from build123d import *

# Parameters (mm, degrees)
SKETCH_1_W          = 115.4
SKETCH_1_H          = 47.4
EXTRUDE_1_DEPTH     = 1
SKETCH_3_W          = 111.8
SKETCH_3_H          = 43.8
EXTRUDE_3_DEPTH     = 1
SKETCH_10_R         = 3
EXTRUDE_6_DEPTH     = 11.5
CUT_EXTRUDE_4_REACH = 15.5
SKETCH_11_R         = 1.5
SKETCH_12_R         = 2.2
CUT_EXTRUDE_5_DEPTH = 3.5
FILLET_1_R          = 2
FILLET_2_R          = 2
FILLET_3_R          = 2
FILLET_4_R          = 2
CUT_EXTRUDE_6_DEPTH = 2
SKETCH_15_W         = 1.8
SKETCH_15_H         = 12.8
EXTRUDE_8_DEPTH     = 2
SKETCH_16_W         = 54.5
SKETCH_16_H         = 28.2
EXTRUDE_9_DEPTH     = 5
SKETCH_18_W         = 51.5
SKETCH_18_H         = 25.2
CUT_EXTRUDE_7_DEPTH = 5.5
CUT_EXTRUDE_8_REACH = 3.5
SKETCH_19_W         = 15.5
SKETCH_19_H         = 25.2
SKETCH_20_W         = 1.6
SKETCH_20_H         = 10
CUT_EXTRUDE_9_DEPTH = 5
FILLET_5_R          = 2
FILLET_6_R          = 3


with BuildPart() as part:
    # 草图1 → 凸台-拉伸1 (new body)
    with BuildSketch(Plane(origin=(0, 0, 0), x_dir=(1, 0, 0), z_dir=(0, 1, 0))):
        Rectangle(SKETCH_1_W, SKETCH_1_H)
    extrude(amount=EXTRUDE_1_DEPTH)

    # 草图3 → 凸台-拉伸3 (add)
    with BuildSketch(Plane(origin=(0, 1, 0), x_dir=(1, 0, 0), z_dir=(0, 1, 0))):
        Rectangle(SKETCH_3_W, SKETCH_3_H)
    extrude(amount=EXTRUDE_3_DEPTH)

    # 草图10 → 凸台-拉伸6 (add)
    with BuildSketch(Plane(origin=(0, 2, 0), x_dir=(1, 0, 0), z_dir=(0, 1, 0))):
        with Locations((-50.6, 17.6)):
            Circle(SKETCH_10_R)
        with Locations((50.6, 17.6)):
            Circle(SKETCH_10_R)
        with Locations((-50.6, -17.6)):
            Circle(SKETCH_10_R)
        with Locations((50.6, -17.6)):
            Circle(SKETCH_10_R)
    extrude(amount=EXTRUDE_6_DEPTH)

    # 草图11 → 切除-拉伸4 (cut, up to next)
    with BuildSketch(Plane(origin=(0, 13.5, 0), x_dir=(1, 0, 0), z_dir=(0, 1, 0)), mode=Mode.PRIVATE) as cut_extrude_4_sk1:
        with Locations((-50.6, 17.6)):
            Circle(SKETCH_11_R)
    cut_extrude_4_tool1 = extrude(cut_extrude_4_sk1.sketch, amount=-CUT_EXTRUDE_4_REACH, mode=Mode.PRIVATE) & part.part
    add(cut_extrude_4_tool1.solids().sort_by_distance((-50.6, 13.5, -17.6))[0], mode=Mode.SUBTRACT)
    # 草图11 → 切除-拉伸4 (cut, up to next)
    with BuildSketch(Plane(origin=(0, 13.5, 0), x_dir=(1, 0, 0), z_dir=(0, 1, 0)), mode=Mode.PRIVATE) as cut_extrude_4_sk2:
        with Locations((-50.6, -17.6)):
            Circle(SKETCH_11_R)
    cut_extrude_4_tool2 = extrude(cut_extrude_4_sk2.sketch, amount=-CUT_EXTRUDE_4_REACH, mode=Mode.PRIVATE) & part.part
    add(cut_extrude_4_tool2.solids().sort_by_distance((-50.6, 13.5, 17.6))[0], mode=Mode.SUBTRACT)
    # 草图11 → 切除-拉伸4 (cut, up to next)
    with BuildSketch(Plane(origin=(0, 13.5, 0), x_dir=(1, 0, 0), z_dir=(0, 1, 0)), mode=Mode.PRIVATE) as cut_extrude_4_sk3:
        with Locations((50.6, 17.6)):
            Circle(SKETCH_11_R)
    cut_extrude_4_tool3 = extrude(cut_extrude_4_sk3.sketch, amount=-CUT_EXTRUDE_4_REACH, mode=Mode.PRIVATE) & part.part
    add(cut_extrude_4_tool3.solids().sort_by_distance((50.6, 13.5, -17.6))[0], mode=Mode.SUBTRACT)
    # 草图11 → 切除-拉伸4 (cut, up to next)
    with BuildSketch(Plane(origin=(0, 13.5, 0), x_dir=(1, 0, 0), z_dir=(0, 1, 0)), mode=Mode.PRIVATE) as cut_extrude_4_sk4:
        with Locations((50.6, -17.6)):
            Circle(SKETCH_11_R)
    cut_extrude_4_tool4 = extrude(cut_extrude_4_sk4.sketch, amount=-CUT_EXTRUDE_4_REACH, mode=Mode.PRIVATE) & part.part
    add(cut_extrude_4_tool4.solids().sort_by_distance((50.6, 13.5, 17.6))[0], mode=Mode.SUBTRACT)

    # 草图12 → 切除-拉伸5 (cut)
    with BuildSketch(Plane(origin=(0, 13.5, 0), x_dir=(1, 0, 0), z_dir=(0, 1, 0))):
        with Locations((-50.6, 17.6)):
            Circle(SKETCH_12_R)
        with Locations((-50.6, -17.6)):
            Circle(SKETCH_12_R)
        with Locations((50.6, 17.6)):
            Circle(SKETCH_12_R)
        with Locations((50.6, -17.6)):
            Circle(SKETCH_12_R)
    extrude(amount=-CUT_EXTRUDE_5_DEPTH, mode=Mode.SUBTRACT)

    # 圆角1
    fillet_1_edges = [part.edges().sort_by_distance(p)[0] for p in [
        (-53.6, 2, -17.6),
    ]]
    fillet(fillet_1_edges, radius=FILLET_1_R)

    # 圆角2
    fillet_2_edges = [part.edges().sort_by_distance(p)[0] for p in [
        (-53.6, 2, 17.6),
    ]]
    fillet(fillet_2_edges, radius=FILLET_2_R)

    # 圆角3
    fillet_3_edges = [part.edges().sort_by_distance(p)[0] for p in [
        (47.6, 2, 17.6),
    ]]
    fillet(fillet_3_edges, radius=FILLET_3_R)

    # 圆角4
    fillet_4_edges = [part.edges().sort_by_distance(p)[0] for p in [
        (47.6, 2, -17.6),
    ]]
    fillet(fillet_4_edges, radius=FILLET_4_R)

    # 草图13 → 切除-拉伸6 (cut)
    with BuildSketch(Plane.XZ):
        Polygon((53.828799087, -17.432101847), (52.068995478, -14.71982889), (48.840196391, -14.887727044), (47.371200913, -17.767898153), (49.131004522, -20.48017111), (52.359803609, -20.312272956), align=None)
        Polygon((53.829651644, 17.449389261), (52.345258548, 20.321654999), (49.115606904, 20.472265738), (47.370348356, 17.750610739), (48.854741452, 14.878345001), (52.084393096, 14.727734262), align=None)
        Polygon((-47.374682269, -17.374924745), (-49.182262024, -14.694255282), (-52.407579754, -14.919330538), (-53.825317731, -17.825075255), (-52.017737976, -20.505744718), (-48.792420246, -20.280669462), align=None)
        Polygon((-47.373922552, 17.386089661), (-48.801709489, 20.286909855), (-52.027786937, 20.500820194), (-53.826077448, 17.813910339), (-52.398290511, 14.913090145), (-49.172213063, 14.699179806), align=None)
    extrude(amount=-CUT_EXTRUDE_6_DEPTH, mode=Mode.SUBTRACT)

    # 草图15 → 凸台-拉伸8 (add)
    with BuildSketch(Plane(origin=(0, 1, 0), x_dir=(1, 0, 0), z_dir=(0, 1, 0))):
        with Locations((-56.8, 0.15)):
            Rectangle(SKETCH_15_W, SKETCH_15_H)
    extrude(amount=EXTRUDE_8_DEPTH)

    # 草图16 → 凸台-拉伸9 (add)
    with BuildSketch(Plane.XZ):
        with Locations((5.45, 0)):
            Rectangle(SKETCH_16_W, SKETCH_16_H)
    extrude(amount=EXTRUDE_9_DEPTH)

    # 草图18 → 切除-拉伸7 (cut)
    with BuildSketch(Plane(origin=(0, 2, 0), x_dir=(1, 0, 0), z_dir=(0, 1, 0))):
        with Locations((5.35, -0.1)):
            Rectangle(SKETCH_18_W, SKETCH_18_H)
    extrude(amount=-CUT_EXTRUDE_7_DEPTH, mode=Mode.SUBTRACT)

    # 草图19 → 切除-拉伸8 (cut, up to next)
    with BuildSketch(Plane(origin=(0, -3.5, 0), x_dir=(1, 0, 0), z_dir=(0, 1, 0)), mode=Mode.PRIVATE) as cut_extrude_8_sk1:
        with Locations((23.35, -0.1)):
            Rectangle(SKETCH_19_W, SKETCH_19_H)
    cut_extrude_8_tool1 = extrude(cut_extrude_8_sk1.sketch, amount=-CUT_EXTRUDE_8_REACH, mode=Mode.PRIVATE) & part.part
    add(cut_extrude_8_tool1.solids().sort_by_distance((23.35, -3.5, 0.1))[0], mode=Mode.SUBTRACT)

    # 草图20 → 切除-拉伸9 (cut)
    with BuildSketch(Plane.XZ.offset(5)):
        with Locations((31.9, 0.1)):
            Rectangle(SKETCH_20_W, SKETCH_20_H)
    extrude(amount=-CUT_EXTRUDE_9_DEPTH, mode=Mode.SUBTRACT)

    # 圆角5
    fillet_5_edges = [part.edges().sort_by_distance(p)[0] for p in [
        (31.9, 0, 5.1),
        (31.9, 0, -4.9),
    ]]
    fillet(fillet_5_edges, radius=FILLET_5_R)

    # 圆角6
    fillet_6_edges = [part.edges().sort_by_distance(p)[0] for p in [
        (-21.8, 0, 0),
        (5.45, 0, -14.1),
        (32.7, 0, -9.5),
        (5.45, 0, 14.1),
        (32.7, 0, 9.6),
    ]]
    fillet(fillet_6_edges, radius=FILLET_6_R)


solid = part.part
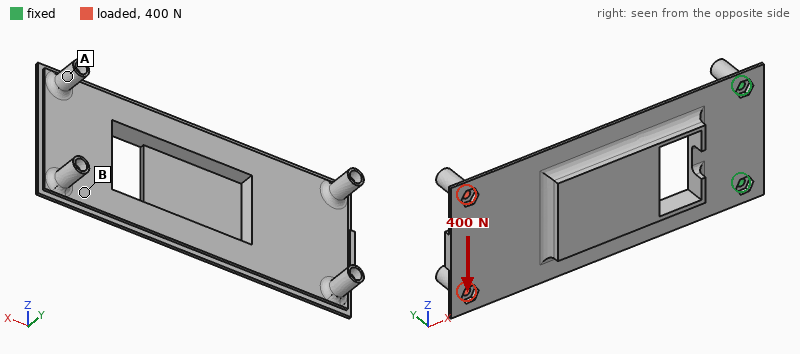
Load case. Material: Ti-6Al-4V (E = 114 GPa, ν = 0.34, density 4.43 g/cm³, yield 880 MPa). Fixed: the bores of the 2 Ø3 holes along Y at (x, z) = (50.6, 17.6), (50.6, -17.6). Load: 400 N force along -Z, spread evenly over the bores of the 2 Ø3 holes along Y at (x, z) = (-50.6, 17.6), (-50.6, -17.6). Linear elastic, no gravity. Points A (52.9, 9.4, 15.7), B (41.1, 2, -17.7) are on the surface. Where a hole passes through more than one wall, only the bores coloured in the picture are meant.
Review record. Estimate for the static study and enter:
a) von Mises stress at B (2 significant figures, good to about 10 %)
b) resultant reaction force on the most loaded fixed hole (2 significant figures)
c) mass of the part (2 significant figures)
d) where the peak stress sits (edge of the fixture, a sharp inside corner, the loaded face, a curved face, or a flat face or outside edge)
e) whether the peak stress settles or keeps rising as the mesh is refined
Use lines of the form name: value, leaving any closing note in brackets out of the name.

von Mises stress at B: 41 MPa
resultant reaction force on the most loaded fixed hole: 1.1 kN
mass of the part: 50 g
where the peak stress sits: edge of the fixture
whether the peak stress settles or keeps rising as the mesh is refined: keeps rising
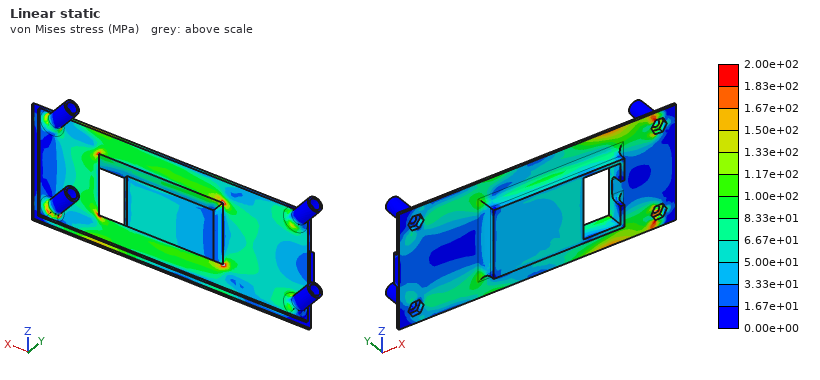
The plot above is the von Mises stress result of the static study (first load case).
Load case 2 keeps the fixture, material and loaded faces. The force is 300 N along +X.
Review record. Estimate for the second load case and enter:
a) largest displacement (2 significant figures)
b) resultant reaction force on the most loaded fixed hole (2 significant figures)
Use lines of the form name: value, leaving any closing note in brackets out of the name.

largest displacement: 1.4 mm
resultant reaction force on the most loaded fixed hole: 150 N
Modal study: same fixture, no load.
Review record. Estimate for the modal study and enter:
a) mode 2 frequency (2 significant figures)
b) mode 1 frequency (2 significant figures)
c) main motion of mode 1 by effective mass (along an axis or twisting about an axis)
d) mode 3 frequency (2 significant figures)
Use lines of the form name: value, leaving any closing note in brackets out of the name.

mode 2 frequency: 750 Hz
mode 1 frequency: 160 Hz
main motion of mode 1 by effective mass: along Y
mode 3 frequency: 1400 Hz
